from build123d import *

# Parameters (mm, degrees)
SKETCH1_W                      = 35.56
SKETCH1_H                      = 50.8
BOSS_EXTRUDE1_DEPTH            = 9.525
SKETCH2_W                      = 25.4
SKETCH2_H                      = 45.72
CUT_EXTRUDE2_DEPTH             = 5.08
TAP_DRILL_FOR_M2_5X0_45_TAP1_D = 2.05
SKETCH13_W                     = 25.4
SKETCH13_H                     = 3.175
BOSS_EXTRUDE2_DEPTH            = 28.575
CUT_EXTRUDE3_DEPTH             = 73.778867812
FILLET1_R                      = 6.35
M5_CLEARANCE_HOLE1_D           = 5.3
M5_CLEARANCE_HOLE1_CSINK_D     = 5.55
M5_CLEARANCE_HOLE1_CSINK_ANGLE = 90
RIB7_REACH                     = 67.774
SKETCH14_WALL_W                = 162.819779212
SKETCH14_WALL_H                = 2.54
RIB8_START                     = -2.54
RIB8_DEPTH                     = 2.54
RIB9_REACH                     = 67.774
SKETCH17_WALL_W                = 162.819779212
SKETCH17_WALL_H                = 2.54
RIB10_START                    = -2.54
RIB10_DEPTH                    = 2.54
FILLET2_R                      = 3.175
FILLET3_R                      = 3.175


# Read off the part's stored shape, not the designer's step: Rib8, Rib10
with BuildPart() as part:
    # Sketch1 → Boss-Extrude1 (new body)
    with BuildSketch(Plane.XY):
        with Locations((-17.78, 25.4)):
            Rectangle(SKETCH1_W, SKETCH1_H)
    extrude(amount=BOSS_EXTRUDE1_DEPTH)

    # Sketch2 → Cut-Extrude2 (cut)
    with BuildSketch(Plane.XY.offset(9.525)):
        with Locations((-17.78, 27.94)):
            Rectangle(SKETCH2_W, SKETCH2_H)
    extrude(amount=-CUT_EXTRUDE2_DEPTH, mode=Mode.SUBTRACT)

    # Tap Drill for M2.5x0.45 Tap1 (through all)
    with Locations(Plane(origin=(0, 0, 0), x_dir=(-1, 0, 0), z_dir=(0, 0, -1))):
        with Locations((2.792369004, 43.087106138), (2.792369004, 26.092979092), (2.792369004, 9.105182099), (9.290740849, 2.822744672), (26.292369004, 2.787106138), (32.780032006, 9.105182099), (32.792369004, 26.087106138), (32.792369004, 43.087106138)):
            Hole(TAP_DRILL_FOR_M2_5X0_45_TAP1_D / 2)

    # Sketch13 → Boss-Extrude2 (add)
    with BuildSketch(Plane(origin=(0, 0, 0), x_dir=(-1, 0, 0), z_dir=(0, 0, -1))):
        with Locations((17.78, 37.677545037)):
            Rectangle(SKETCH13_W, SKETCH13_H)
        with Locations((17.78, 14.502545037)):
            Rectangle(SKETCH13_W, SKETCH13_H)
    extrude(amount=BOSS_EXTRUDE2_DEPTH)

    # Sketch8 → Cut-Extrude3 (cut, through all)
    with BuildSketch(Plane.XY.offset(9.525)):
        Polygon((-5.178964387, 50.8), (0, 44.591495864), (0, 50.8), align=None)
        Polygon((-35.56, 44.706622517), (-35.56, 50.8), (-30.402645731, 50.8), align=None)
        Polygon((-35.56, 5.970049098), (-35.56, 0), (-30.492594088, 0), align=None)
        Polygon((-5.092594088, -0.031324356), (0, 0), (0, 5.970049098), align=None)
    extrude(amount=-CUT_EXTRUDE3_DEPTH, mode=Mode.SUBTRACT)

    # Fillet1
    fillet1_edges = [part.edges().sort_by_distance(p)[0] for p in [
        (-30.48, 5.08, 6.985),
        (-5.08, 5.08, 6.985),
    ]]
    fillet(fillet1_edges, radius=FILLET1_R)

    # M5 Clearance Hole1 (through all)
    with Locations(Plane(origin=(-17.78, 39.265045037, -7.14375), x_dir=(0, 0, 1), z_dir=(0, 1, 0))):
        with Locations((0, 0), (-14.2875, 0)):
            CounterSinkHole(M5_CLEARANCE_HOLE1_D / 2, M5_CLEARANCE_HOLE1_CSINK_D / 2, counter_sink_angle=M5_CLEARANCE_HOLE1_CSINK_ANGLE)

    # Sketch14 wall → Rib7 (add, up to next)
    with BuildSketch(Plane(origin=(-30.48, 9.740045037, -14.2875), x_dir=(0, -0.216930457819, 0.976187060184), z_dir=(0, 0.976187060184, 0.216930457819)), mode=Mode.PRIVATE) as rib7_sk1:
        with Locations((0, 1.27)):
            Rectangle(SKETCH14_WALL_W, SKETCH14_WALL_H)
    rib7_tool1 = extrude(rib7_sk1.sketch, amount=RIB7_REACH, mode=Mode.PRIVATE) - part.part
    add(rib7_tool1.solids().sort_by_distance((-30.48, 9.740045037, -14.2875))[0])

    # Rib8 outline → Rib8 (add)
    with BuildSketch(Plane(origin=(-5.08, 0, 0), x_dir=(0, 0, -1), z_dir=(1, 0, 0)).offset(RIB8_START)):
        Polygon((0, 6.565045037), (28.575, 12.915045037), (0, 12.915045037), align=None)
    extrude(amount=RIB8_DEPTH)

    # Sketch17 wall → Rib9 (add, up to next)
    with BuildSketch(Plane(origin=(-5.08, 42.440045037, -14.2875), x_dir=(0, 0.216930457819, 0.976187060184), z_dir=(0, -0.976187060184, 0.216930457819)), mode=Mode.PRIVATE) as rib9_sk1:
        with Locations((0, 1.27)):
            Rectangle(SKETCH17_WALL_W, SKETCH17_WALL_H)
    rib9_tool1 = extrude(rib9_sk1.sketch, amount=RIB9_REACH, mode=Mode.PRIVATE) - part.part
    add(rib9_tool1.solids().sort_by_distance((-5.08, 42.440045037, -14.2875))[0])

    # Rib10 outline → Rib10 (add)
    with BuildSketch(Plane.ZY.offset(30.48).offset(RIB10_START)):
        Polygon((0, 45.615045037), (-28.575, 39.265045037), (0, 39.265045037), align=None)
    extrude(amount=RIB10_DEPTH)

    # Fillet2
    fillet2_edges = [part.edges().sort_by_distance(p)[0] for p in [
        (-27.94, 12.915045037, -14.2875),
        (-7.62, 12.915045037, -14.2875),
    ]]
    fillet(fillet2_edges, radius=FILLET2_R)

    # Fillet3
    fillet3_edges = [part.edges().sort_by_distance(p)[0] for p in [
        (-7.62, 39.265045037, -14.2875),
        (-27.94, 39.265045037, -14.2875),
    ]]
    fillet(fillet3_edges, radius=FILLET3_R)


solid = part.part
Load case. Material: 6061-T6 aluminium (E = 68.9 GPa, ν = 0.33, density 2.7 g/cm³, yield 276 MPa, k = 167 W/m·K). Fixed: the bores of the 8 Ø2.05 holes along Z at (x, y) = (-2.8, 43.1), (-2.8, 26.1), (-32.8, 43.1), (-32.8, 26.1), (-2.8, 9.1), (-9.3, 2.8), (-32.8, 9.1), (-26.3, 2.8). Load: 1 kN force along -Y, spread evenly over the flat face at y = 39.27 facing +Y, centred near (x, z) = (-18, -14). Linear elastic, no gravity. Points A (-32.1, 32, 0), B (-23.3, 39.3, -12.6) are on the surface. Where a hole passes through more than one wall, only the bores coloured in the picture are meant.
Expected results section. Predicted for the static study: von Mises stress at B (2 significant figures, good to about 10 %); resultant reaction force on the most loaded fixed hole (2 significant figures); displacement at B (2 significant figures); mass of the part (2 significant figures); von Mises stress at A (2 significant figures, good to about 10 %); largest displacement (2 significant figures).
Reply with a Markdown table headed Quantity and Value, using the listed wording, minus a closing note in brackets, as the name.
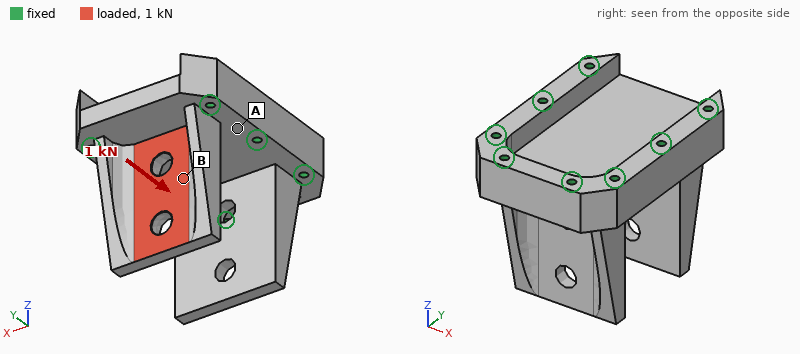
| Quantity | Value |
|---|---|
| von Mises stress at B | 33 MPa |
| resultant reaction force on the most loaded fixed hole | 500 N |
| displacement at B | 0.060 mm |
| mass of the part | 43 g |
| von Mises stress at A | 13 MPa |
| largest displacement | 0.19 mm |
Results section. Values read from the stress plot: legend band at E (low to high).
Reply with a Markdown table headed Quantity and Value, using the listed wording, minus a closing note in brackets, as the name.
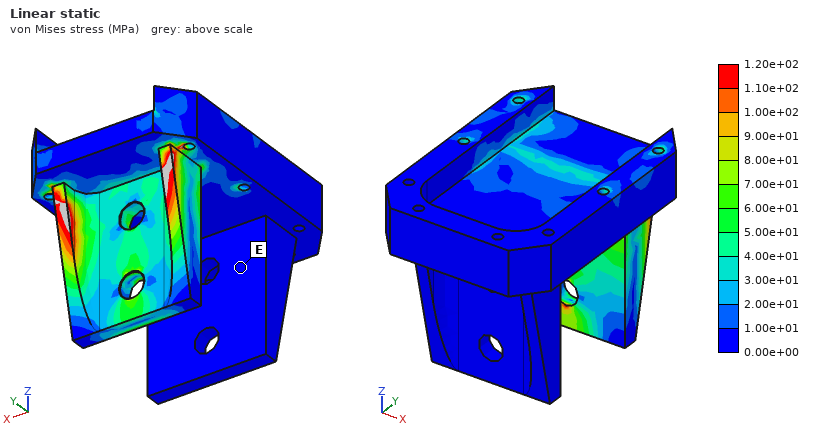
| Quantity | Value |
|---|---|
| legend band at E | 0.00e+00 to 1.00e+01 MPa |
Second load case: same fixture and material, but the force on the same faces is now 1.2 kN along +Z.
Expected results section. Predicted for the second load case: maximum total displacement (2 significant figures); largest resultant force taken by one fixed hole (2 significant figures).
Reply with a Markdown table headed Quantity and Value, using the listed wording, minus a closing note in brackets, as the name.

| Quantity | Value |
|---|---|
| maximum total displacement | 14 µm |
| largest resultant force taken by one fixed hole | 480 N |
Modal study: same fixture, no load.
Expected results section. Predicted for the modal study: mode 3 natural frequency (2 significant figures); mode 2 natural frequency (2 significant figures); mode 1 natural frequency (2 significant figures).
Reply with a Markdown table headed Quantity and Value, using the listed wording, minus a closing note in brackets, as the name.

| Quantity | Value |
|---|---|
| mode 3 natural frequency | 10 kHz |
| mode 2 natural frequency | 6100 Hz |
| mode 1 natural frequency | 5900 Hz |
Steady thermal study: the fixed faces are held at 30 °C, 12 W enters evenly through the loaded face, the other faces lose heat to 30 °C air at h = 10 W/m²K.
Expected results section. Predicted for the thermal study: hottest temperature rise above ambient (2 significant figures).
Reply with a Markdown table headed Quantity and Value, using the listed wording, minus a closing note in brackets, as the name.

| Quantity | Value |
|---|---|
| hottest temperature rise above ambient | 15 K |
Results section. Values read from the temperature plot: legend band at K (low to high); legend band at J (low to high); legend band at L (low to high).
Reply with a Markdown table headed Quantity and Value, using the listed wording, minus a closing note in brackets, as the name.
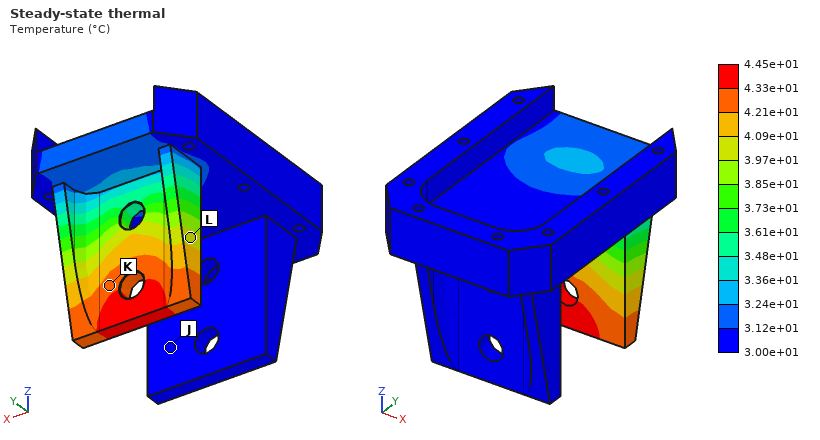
| Quantity | Value |
|---|---|
| legend band at K | 4.21e+01 to 4.33e+01 °C |
| legend band at J | 3.00e+01 to 3.12e+01 °C |
| legend band at L | 3.97e+01 to 4.09e+01 °C |
